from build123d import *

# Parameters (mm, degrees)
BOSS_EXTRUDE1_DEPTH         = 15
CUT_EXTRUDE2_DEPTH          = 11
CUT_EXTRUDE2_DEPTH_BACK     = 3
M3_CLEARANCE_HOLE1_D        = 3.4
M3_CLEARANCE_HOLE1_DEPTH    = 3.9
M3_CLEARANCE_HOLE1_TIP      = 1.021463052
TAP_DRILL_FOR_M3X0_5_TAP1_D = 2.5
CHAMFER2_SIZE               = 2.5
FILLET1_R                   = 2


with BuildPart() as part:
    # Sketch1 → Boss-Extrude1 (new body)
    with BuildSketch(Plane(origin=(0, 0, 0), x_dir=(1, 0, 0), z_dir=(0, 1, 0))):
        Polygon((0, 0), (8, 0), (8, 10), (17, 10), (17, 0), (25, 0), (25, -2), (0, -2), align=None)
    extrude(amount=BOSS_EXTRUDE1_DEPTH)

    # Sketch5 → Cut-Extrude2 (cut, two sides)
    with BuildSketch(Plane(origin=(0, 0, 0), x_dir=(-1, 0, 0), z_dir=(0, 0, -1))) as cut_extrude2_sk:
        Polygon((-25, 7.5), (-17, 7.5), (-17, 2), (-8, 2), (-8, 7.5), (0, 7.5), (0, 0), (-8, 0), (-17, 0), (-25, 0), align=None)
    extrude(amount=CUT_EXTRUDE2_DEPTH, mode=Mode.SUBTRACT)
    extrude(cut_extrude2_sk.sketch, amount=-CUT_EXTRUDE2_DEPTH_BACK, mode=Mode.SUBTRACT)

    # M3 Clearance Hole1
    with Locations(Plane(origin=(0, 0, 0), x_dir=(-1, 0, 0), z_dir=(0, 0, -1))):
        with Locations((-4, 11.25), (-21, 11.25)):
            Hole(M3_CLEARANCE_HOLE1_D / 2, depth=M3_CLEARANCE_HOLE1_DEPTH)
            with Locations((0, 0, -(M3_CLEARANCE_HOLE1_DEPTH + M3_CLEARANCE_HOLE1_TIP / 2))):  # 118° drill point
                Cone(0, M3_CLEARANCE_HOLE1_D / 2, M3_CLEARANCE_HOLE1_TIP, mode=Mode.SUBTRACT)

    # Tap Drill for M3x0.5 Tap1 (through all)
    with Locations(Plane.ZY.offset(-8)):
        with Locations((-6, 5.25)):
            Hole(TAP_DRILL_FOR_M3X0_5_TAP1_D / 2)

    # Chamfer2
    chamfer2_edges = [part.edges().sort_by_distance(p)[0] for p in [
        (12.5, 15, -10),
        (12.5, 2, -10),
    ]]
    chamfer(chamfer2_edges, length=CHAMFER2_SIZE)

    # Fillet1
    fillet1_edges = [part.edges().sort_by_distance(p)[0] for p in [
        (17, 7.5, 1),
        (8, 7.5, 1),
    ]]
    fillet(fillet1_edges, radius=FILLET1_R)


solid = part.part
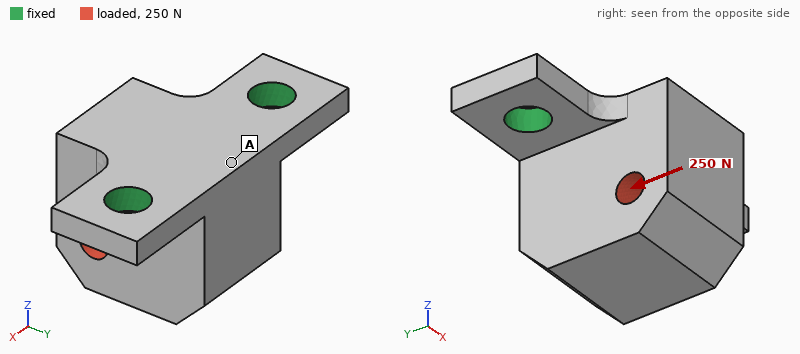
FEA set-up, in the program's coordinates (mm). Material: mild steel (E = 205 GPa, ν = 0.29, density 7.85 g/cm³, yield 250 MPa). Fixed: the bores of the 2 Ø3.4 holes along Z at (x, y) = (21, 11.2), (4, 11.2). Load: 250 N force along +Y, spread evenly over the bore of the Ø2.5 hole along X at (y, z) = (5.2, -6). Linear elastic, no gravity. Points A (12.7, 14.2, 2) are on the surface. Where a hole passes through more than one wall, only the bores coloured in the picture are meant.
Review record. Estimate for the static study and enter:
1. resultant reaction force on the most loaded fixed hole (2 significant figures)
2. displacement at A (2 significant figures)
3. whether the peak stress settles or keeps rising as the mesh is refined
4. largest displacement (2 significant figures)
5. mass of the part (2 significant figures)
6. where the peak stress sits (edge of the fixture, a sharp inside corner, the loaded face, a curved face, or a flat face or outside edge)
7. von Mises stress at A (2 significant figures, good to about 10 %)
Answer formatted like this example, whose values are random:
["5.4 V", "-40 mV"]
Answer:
["130 N", "4.4 µm", "keeps rising", "19 µm", "12 g", "edge of the fixture", "20 MPa"]
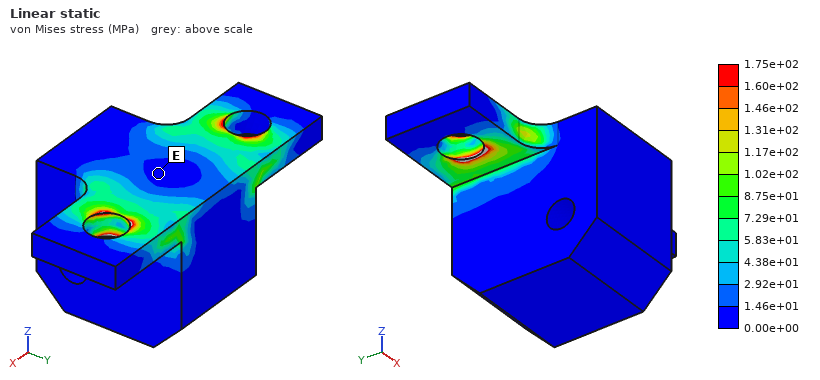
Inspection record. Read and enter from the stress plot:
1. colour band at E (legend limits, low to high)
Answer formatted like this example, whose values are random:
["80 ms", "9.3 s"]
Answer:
["0.00e+00 to 1.46e+01 MPa"]
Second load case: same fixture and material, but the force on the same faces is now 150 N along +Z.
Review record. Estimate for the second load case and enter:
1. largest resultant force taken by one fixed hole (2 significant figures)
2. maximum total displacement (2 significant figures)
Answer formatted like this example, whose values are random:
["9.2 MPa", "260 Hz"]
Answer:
["80 N", "9.7 µm"]
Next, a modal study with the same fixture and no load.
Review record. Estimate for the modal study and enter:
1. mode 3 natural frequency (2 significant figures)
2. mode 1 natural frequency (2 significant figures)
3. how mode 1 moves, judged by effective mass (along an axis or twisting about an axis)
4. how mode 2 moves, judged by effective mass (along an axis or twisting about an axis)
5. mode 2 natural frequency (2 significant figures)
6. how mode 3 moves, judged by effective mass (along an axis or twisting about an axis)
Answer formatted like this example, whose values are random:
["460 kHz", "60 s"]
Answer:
["24 kHz", "7400 Hz", "along Y", "along X", "20 kHz", "along Z"]
